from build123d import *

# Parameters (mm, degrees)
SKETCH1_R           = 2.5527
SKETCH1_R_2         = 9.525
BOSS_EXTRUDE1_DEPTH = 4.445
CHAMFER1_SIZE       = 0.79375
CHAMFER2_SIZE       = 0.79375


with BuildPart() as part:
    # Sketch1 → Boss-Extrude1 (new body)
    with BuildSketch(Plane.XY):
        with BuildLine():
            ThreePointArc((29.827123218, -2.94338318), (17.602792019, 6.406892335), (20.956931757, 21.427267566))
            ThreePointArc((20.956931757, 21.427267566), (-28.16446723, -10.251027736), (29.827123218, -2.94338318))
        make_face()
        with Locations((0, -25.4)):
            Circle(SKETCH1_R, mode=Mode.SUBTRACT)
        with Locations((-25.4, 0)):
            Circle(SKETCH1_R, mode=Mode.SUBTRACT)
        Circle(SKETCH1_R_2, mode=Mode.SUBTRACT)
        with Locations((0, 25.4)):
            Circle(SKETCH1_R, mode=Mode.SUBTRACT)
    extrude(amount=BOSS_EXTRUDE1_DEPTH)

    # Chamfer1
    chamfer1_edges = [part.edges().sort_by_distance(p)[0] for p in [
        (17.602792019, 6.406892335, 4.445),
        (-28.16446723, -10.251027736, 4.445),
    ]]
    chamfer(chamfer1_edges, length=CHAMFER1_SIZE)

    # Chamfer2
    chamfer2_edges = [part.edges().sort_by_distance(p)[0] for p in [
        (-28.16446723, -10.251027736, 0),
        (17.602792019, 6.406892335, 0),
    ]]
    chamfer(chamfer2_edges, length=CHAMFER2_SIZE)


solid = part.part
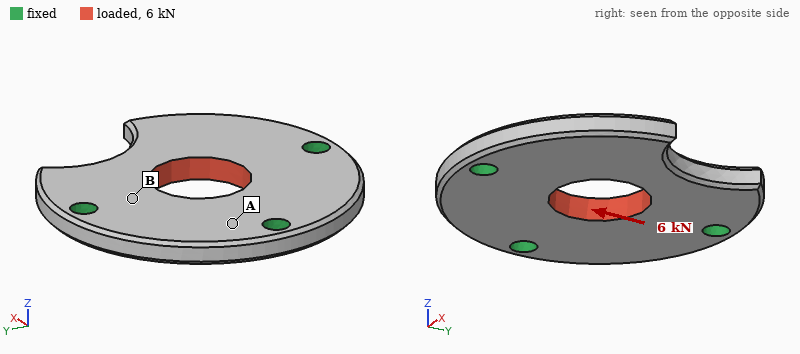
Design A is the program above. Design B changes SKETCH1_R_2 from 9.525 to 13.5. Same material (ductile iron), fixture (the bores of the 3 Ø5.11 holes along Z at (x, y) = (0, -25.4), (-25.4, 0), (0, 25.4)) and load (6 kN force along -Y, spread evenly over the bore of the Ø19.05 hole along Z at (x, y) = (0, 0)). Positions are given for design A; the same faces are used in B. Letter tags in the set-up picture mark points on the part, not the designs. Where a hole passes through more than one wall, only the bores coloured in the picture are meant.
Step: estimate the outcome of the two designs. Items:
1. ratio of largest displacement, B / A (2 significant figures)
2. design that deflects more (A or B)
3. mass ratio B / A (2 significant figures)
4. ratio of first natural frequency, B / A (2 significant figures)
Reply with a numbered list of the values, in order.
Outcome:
1. 1.5
2. B
3. 0.87
4. 0.95
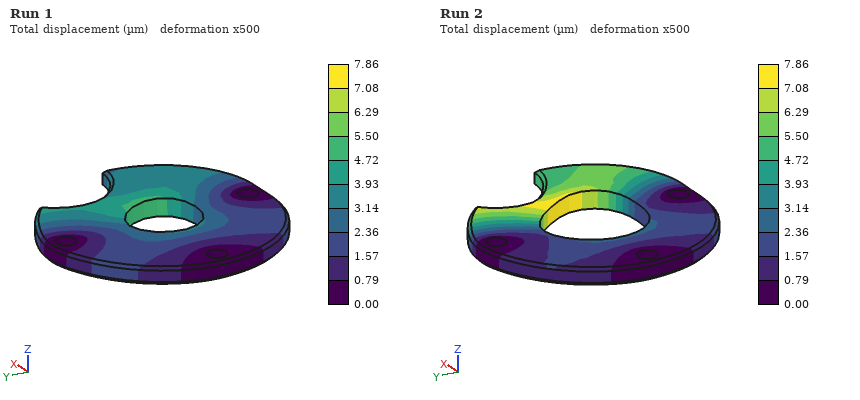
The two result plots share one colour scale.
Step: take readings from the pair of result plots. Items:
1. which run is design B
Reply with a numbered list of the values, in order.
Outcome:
1. Run 2
